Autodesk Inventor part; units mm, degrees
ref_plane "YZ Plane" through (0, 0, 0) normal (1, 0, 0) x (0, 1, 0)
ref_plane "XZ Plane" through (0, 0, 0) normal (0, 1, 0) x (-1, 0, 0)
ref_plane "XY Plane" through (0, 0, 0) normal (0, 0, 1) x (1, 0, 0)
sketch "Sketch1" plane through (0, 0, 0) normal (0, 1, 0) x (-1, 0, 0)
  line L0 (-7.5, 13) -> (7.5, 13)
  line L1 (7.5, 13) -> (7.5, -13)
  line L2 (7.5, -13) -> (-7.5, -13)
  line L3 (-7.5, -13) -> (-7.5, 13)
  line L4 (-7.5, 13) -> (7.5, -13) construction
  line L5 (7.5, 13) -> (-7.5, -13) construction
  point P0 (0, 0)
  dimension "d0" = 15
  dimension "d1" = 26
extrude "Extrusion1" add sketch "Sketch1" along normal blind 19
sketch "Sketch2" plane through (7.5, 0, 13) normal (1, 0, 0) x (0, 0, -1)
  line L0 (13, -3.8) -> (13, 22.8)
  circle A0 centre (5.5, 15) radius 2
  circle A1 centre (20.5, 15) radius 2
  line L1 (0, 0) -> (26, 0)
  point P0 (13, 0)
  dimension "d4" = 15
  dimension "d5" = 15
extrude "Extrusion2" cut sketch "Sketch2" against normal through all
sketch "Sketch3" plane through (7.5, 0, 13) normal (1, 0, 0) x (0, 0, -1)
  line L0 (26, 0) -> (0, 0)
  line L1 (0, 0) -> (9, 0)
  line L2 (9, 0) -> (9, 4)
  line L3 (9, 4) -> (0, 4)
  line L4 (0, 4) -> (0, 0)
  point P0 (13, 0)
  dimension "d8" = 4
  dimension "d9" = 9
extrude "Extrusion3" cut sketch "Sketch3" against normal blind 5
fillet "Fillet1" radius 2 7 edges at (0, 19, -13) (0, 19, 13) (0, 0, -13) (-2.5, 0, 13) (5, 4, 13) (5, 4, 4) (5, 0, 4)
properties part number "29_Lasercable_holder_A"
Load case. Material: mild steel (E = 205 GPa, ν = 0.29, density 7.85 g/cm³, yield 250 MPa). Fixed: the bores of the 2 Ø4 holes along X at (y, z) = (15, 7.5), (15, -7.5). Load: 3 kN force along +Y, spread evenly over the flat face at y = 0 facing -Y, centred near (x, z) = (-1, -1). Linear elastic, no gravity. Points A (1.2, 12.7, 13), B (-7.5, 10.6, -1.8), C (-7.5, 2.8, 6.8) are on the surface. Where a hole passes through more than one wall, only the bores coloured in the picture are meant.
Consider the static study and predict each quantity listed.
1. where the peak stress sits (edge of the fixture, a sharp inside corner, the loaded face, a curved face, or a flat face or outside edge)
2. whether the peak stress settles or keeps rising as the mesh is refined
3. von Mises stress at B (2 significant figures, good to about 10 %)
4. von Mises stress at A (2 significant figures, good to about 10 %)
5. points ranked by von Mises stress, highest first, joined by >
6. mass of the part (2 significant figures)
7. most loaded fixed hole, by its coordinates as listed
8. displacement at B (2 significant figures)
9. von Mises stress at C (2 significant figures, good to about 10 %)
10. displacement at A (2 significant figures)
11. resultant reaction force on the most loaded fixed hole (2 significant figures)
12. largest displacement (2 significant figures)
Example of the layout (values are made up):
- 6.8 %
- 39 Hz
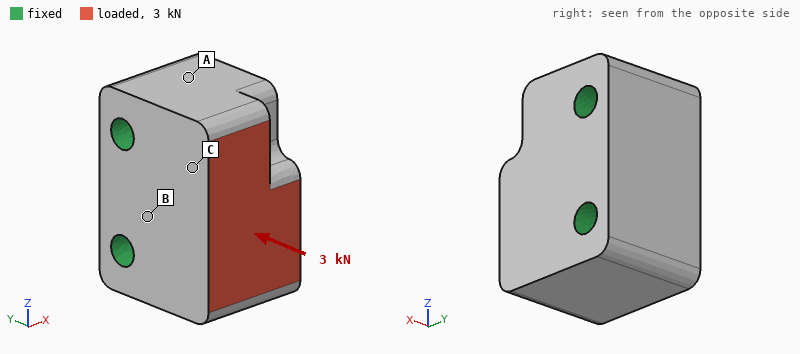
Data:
- edge of the fixture
- keeps rising
- 7.3 MPa
- 2.7 MPa
- C > B > A
- 53 g
- (15, -7.5)
- 0.38 µm
- 11 MPa
- 0.14 µm
- 1.7 kN
- 0.92 µm
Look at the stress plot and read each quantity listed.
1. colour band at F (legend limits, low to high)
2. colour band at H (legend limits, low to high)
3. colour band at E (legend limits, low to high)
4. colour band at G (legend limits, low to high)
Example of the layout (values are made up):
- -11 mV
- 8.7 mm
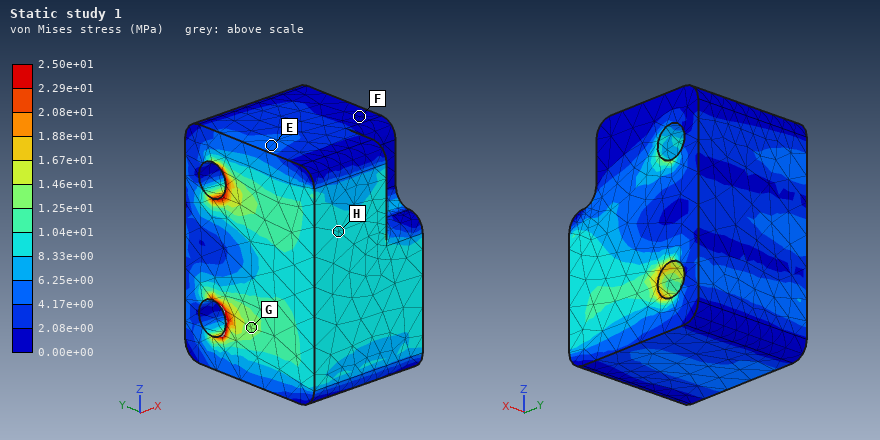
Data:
- 0.00e+00 to 2.08e+00 MPa
- 8.33e+00 to 1.04e+01 MPa
- 4.17e+00 to 6.25e+00 MPa
- 1.25e+01 to 1.46e+01 MPa
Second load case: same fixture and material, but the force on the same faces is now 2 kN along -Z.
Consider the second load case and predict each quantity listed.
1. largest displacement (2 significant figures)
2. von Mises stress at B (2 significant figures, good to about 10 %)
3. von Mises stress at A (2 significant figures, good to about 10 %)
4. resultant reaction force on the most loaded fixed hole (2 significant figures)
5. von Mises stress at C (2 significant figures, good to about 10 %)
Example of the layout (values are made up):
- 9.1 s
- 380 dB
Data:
- 2.0 µm
- 13 MPa
- 10 MPa
- 1.9 kN
- 11 MPa
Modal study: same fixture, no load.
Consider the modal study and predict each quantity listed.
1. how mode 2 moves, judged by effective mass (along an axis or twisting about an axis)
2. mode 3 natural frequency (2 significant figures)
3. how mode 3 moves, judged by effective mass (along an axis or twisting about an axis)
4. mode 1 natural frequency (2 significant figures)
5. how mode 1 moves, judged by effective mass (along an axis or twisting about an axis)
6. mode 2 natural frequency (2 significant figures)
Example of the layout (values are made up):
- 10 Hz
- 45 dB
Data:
- along Z
- 51 kHz
- twisting about Y
- 36 kHz
- along X
- 43 kHz
